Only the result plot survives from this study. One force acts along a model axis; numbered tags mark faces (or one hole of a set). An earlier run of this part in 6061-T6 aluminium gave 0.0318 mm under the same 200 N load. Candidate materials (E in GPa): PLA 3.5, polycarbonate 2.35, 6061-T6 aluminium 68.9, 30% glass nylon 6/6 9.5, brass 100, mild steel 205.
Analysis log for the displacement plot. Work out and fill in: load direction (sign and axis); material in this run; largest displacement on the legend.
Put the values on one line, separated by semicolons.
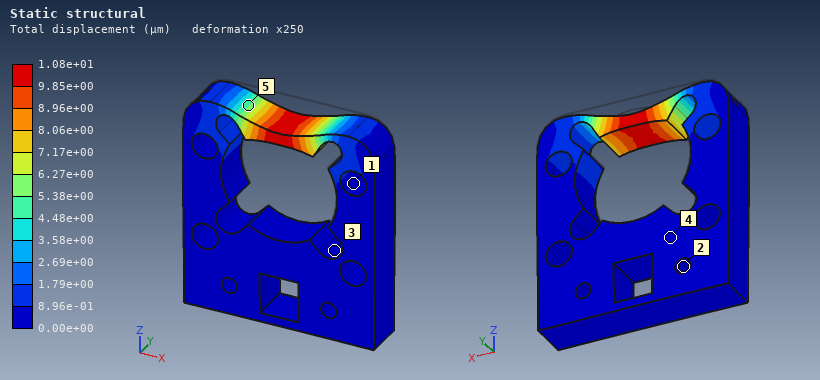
-Z; mild steel; 1.08e+01 µm
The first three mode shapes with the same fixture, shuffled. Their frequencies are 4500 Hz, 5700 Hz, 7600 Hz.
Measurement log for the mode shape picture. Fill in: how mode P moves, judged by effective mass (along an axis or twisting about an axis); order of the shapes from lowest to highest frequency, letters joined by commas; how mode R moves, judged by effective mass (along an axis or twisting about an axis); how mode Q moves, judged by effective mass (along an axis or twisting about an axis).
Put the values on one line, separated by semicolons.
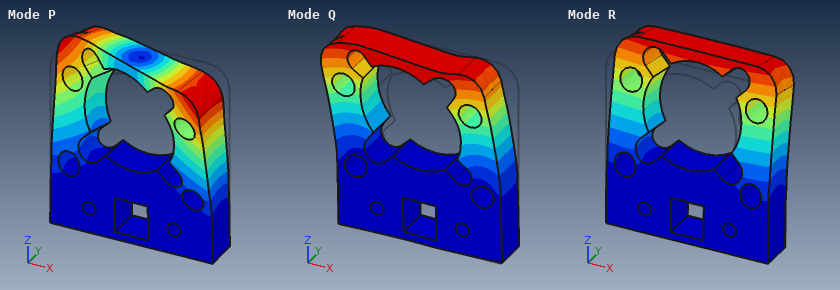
twisting about Z; R, Q, P; along Y; along X
